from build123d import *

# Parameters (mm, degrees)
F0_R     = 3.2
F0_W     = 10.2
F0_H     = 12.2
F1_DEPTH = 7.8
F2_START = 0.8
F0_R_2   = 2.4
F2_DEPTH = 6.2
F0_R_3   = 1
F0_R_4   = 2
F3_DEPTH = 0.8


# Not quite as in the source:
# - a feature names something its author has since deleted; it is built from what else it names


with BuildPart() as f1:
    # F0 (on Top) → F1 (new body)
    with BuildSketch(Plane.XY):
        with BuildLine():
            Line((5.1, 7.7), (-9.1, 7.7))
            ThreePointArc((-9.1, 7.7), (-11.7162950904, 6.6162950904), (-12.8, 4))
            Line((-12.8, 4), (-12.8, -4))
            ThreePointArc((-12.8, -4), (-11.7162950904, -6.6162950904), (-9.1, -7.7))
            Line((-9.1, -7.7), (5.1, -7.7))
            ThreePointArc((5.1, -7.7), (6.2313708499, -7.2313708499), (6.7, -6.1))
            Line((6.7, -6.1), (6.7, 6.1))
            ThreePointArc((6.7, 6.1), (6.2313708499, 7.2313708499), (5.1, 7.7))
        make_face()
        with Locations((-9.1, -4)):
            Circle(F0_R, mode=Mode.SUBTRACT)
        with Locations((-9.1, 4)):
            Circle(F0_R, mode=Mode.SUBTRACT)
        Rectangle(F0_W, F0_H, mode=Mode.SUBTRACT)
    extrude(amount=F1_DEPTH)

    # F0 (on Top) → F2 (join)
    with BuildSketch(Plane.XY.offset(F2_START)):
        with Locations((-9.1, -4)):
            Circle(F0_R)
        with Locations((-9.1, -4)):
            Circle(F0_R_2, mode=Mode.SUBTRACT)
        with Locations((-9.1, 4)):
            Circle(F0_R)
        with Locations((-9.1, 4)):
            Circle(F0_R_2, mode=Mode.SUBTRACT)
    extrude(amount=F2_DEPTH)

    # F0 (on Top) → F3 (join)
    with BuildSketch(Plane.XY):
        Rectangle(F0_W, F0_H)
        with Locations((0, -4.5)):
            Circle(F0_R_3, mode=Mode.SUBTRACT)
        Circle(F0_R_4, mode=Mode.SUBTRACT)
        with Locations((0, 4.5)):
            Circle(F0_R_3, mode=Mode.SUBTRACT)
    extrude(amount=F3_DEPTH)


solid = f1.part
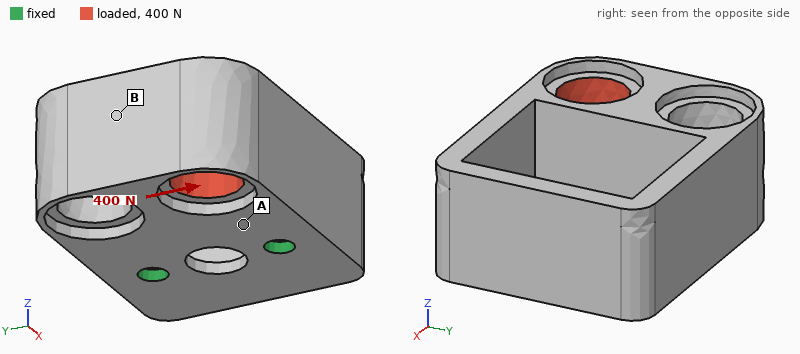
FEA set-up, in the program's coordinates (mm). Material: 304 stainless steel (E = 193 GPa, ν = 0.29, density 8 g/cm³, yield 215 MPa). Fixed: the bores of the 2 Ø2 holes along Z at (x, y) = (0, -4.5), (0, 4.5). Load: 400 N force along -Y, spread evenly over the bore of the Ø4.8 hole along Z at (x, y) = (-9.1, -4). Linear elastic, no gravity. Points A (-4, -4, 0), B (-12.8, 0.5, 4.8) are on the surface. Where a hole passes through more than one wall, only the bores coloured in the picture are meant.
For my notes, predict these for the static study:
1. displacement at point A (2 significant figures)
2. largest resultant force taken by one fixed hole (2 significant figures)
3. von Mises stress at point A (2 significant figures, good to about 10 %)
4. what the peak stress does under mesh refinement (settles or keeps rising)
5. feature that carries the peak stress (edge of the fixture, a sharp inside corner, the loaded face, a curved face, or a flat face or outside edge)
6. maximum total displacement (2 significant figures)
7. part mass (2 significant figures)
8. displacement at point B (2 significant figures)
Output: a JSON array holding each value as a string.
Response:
["3.5 µm", "400 N", "53 MPa", "keeps rising", "edge of the fixture", "13 µm", "8.6 g", "9.8 µm"]
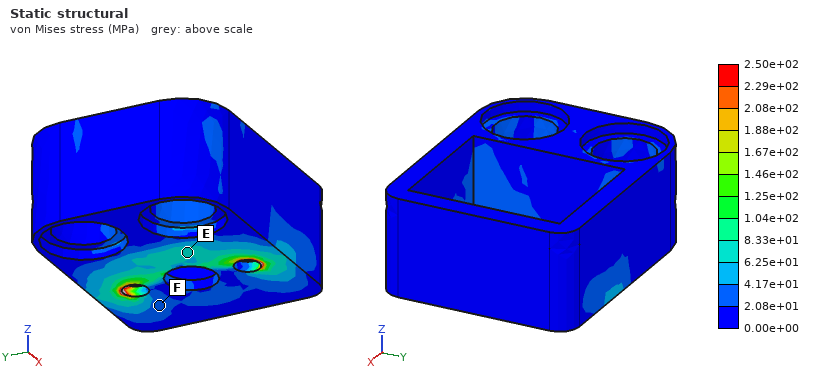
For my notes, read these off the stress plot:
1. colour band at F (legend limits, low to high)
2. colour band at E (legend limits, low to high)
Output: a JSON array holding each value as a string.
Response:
["2.08e+01 to 4.17e+01 MPa", "6.25e+01 to 8.33e+01 MPa"]
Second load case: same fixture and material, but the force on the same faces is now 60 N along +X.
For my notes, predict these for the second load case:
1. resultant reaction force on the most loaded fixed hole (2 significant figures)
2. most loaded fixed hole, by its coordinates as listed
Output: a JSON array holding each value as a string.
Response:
["54 N", "(0, -4.5)"]
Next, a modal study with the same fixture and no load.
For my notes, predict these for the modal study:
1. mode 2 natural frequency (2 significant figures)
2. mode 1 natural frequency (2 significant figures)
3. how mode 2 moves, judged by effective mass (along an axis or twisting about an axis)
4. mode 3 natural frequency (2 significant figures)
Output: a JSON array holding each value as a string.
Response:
["14 kHz", "3800 Hz", "along Y", "18 kHz"]
